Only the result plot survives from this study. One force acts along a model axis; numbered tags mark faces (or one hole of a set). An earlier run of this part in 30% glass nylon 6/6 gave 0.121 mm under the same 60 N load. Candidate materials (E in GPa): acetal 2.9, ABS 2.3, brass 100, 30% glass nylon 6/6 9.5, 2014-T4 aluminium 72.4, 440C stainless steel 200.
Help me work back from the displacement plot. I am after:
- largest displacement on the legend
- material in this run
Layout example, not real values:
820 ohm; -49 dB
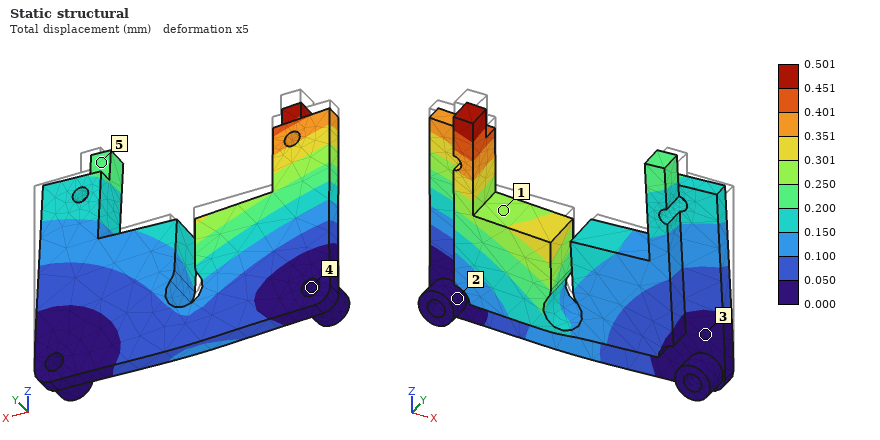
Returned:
0.501 mm; ABS
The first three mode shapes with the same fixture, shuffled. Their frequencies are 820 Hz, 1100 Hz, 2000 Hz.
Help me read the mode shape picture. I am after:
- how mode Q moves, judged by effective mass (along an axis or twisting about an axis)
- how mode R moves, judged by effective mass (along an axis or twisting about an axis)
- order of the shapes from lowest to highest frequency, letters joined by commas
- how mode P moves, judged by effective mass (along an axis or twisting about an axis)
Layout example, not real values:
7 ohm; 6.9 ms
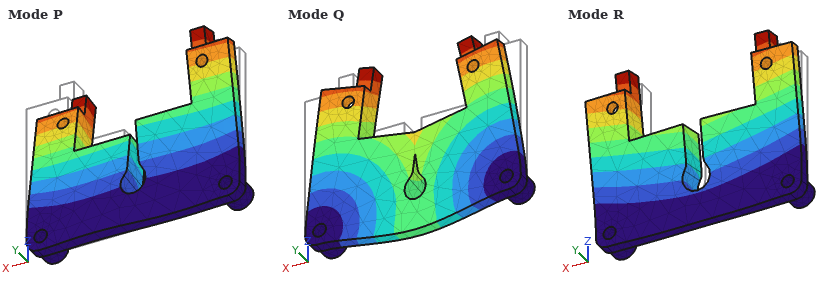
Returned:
along Z; along Y; R, P, Q; twisting about Z
